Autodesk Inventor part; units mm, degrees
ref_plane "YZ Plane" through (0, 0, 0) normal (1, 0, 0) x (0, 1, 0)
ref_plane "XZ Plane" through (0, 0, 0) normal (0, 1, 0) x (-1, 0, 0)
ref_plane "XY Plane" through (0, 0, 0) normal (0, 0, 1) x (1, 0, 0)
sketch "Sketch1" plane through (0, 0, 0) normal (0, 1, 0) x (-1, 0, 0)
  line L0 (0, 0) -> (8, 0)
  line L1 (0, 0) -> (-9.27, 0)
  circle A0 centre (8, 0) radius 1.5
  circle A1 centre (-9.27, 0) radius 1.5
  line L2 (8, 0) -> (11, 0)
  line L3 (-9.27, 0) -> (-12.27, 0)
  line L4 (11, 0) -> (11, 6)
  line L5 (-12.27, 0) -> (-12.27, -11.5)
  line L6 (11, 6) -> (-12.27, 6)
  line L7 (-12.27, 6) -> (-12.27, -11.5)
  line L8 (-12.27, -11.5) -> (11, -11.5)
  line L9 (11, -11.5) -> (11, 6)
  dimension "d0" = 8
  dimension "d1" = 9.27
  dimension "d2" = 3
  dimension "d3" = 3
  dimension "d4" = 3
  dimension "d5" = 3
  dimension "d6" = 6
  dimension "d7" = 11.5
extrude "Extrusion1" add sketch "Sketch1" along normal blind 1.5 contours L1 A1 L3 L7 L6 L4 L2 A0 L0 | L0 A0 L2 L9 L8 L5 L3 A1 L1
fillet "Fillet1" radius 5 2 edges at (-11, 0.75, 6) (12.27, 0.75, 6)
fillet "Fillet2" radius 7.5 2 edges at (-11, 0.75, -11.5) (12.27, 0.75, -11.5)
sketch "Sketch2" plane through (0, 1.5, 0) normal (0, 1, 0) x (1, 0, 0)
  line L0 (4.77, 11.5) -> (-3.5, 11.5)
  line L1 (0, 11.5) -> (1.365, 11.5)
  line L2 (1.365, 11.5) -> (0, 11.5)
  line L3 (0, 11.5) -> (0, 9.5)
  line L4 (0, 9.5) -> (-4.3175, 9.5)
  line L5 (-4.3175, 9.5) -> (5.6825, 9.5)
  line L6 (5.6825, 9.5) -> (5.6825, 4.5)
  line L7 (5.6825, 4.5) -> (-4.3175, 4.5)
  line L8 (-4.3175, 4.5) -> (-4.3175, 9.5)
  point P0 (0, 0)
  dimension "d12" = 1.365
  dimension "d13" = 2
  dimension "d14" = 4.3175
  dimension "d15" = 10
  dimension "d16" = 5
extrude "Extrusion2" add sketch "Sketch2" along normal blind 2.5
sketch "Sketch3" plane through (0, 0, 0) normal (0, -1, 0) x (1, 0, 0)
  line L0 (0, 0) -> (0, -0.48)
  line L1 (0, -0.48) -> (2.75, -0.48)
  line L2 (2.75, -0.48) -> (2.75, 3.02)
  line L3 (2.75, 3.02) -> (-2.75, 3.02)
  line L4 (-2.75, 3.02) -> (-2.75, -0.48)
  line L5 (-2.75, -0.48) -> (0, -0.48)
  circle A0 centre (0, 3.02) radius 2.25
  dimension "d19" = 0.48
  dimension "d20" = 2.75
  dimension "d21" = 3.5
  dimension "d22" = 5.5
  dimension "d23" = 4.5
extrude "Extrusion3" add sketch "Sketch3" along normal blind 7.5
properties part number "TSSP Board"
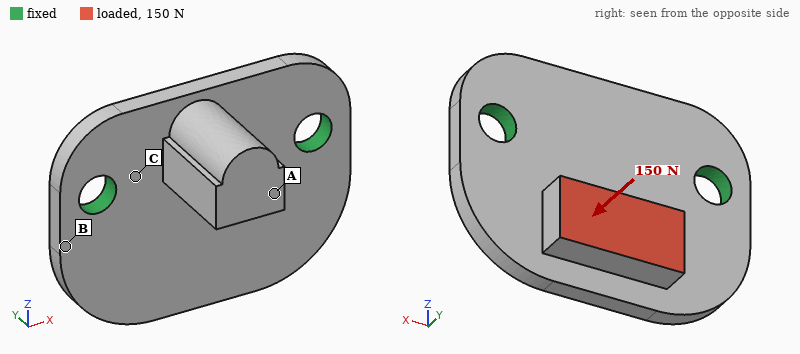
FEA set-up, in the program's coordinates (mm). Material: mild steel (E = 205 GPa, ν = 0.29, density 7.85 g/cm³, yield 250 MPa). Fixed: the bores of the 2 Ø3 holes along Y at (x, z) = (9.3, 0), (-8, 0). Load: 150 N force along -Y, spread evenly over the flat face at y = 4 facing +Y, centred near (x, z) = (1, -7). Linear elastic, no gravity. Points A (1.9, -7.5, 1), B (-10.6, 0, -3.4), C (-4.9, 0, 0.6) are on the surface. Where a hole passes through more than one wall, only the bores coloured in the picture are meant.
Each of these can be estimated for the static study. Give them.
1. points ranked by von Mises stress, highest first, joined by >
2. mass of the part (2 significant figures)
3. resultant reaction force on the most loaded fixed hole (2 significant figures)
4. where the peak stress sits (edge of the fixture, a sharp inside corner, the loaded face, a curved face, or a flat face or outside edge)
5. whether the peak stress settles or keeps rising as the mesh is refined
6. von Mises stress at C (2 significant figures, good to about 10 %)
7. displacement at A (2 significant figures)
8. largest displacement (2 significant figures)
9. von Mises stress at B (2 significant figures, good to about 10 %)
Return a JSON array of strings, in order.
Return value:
["B > C > A", "6.8 g", "76 N", "edge of the fixture", "keeps rising", "40 MPa", "6.6 µm", "26 µm", "75 MPa"]
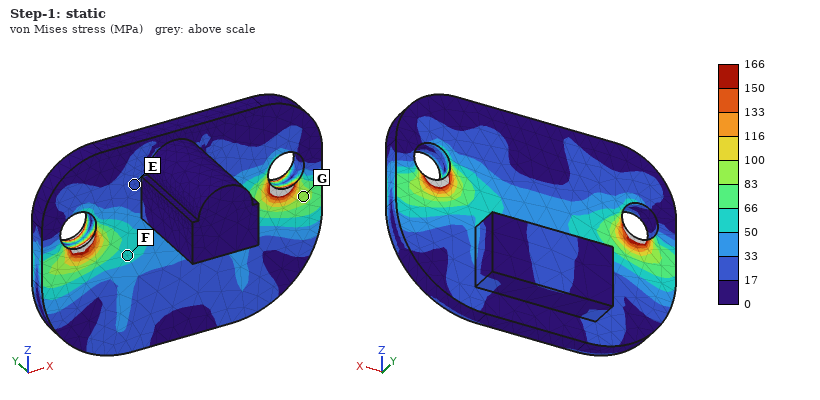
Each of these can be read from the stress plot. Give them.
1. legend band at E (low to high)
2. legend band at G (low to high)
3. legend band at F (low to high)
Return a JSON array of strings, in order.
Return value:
["17 to 33 MPa", "83 to 100 MPa", "50 to 66 MPa"]
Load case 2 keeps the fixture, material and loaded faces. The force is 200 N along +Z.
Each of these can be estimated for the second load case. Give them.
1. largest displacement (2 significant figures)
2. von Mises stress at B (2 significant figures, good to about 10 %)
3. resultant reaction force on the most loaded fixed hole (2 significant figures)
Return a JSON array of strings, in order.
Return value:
["23 µm", "62 MPa", "100 N"]
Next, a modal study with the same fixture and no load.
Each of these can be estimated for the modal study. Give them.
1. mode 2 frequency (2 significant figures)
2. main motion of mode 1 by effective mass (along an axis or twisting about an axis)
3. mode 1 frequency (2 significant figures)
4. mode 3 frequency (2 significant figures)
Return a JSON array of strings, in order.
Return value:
["14 kHz", "along Y", "8700 Hz", "23 kHz"]
